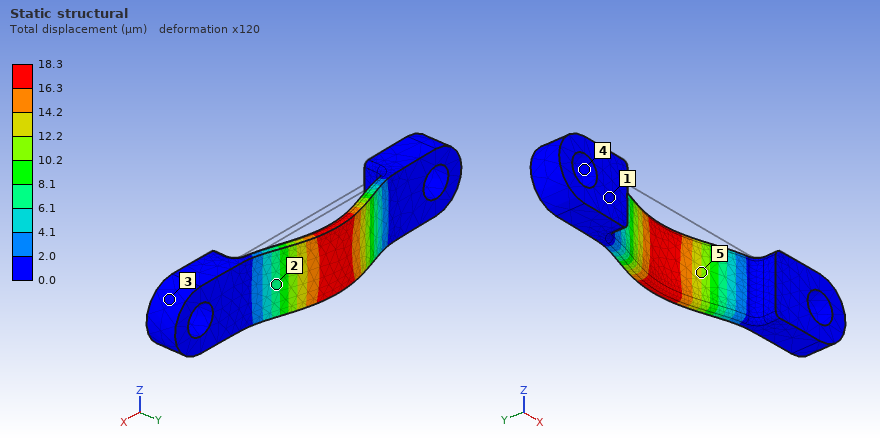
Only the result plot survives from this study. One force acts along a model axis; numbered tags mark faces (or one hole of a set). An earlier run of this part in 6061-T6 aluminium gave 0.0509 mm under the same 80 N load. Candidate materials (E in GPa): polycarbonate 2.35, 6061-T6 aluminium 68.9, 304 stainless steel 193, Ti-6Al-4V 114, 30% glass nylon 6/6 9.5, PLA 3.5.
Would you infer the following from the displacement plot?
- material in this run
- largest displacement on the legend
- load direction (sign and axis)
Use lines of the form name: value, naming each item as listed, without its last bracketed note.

material in this run: 304 stainless steel
largest displacement on the legend: 18.3 µm
load direction: +Y
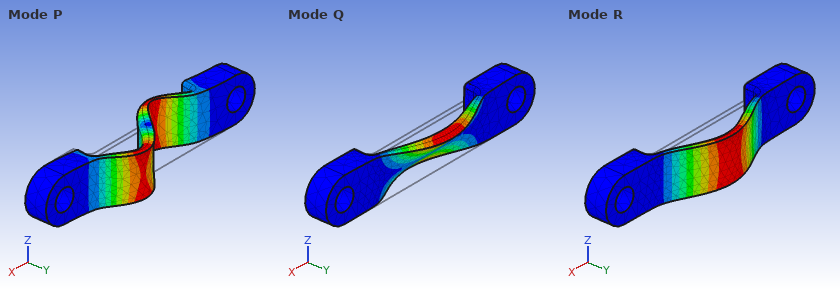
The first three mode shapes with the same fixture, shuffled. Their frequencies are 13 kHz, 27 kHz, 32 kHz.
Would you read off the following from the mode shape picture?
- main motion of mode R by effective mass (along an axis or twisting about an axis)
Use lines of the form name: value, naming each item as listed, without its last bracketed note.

main motion of mode R by effective mass: along Y
